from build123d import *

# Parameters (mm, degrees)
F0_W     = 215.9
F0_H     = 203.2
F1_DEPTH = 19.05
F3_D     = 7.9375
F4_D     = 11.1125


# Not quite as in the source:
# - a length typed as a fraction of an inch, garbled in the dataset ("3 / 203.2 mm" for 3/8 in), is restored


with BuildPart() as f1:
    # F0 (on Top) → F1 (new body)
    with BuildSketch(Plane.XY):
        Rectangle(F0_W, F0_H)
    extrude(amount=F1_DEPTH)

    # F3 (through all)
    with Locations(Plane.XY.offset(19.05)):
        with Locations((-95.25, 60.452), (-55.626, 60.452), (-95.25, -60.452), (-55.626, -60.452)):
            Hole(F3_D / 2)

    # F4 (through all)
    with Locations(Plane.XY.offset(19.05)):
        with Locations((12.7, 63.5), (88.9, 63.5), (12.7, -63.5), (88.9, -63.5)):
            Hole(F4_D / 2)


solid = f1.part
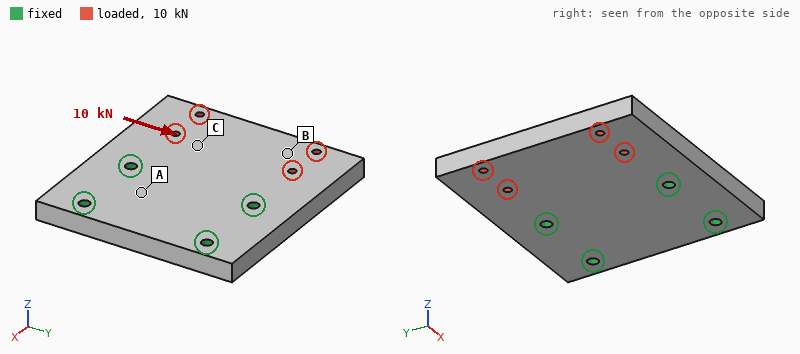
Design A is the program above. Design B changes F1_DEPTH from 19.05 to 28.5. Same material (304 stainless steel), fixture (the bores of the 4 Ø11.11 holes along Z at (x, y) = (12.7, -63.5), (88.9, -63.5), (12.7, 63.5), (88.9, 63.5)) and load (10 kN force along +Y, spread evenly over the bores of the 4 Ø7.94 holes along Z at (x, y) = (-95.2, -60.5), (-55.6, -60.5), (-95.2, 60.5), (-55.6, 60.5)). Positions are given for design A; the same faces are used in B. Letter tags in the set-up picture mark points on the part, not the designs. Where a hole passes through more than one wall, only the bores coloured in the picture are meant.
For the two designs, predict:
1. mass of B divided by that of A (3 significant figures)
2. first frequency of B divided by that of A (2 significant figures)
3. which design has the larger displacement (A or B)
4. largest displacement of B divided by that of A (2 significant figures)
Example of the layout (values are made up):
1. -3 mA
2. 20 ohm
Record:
1. 1.50
2. 1.4
3. A
4. 0.67
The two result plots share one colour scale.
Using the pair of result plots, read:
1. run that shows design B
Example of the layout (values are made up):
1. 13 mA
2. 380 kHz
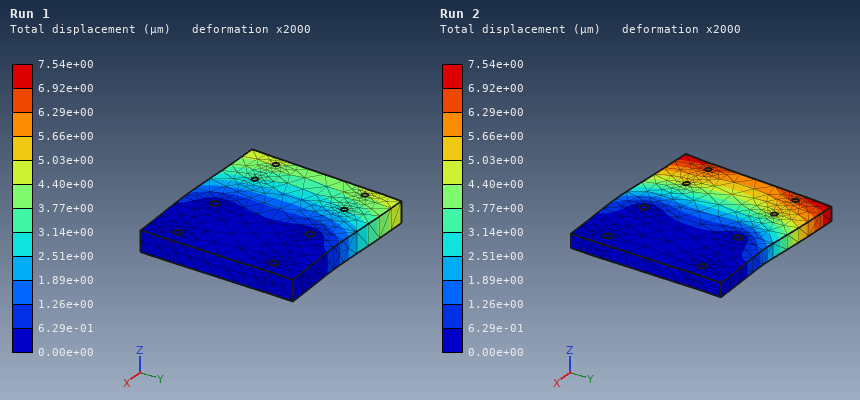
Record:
1. Run 1
